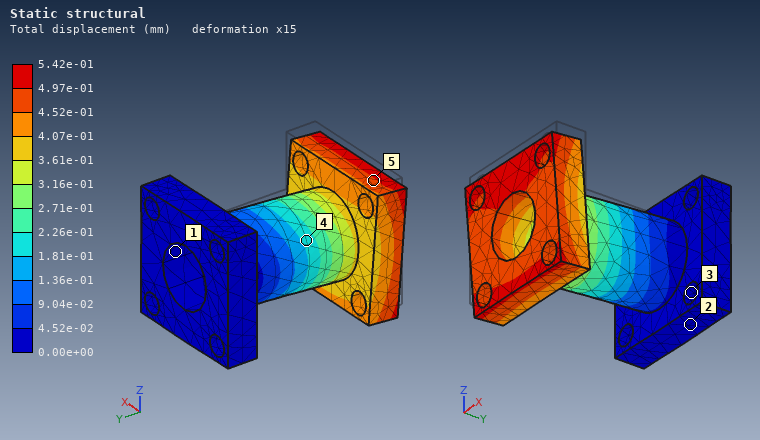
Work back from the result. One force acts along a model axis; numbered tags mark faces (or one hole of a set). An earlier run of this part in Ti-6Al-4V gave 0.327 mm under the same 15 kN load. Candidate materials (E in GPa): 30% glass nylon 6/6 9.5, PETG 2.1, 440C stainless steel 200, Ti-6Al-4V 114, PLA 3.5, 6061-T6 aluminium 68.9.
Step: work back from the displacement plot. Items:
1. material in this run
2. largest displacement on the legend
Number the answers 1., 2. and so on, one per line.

1. 6061-T6 aluminium
2. 5.42e-01 mm
